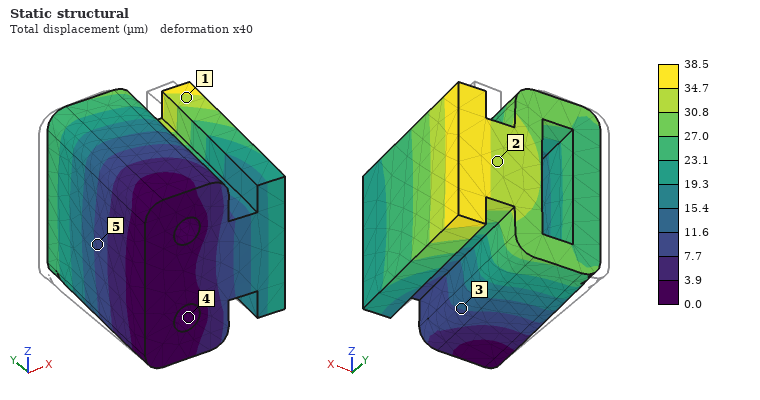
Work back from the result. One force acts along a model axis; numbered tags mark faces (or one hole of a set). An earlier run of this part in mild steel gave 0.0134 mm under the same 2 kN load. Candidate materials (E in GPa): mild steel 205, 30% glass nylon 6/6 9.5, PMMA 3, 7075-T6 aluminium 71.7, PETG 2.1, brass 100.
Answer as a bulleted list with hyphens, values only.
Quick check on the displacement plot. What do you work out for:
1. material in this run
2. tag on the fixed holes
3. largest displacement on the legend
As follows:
- 7075-T6 aluminium
- 4
- 38.5 µm
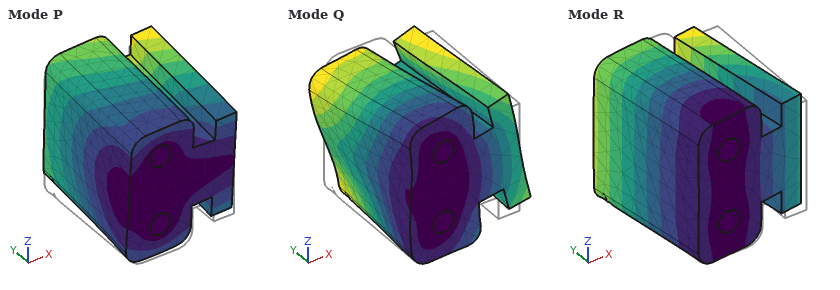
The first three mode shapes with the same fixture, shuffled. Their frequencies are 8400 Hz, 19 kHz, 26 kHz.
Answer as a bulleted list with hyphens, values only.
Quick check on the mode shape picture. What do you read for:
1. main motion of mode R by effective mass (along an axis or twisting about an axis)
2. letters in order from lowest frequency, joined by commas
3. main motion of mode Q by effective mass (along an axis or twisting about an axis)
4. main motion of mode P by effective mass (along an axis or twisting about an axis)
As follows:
- along X
- R, P, Q
- twisting about Y
- along Z
